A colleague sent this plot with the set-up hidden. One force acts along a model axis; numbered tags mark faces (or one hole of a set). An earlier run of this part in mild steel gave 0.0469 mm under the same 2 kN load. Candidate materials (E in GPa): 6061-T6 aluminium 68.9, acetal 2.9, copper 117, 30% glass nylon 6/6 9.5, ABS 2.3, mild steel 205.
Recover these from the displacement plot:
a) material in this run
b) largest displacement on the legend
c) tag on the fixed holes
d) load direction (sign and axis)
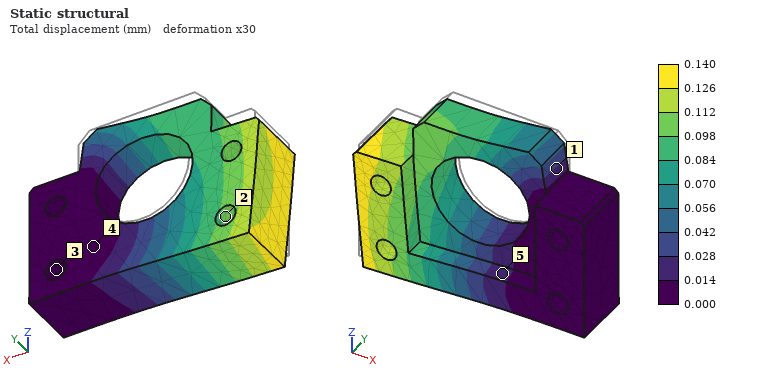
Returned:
6061-T6 aluminium
0.140 mm
3
-Z
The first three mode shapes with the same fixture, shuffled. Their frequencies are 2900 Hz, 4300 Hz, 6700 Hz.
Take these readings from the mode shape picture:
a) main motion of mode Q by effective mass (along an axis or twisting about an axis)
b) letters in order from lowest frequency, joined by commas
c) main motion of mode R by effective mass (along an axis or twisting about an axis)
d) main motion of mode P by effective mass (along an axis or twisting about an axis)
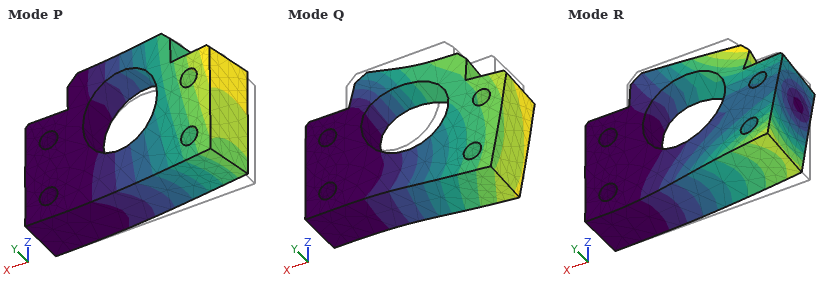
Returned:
along Z
P, Q, R
twisting about X
along Y
